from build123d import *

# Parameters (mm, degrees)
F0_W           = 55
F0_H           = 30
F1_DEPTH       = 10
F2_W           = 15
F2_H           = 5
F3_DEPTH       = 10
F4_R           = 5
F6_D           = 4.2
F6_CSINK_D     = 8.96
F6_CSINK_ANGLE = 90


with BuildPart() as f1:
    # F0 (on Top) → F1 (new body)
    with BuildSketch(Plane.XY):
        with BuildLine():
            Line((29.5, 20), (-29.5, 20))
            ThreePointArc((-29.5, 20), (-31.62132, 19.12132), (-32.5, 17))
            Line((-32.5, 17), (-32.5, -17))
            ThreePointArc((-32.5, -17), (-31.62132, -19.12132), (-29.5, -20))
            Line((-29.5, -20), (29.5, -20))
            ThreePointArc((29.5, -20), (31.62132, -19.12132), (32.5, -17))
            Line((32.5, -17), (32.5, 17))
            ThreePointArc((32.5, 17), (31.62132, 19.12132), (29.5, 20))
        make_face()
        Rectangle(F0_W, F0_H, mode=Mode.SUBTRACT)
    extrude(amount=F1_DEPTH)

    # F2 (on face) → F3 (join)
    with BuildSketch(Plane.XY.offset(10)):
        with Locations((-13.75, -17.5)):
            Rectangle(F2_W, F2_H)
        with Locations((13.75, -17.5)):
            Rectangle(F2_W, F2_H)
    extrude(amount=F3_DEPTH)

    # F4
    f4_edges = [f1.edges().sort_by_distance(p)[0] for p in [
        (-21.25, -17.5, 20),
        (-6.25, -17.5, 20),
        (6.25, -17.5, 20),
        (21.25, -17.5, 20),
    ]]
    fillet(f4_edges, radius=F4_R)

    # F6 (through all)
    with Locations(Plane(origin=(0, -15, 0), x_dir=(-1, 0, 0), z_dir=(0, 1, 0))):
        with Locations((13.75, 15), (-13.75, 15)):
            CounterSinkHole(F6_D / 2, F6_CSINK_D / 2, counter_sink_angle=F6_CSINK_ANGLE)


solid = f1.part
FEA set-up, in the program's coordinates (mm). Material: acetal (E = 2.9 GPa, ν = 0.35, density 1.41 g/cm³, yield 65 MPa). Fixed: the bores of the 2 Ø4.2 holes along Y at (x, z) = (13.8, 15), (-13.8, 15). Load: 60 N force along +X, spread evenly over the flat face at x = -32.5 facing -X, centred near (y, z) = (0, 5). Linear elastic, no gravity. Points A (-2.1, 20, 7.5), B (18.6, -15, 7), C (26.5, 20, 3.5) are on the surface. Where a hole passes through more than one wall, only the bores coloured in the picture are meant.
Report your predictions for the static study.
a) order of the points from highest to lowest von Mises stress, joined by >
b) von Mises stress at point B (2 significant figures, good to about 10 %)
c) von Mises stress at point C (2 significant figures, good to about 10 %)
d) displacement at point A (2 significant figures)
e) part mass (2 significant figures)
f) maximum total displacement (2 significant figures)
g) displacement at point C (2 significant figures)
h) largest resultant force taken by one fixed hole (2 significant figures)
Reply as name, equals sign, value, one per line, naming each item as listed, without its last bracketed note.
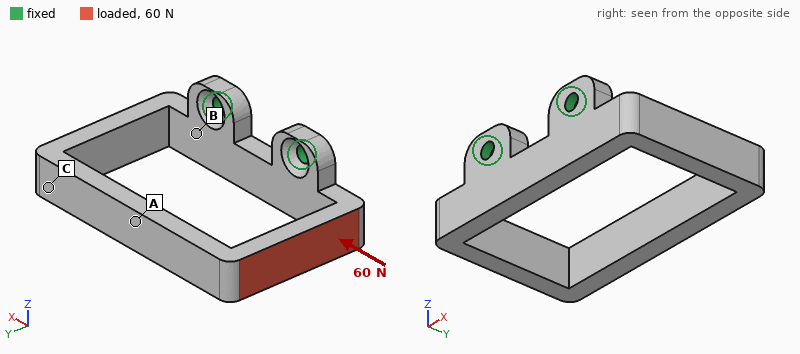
order of the points from highest to lowest von Mises stress, joined by > = B > C > A
von Mises stress at point B = 7.2 MPa
von Mises stress at point C = 4.8 MPa
displacement at point A = 0.79 mm
part mass = 15 g
maximum total displacement = 0.85 mm
displacement at point C = 0.82 mm
largest resultant force taken by one fixed hole = 42 N
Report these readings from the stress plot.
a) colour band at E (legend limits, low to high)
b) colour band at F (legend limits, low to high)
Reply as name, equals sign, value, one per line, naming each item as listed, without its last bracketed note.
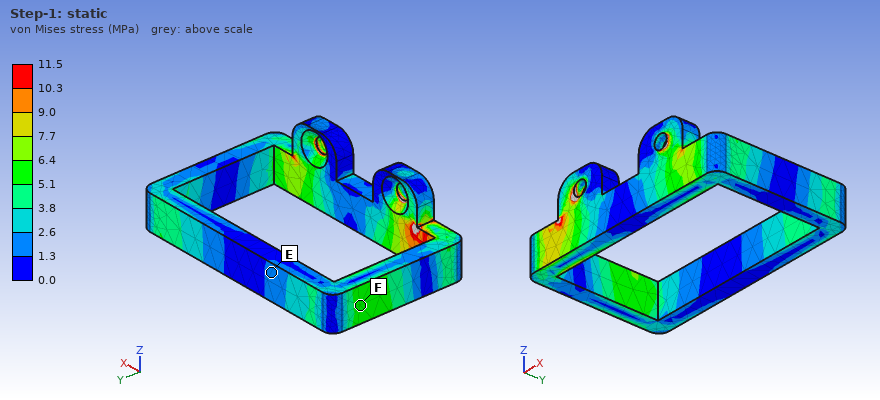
colour band at E = 1.3 to 2.6 MPa
colour band at F = 5.1 to 6.4 MPa
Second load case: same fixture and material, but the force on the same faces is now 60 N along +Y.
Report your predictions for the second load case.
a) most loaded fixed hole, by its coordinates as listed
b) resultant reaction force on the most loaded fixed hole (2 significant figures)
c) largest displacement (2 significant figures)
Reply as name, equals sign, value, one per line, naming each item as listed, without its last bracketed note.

most loaded fixed hole, by its coordinates as listed = (-13.8, 15)
resultant reaction force on the most loaded fixed hole = 80 N
largest displacement = 0.81 mm
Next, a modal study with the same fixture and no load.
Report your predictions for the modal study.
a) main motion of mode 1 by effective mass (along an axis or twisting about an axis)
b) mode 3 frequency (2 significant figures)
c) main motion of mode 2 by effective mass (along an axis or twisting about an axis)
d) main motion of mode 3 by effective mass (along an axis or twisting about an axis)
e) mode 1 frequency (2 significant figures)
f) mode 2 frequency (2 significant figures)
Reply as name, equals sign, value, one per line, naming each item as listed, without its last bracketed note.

main motion of mode 1 by effective mass = along Z
mode 3 frequency = 680 Hz
main motion of mode 2 by effective mass = along X
main motion of mode 3 by effective mass = twisting about Y
mode 1 frequency = 310 Hz
mode 2 frequency = 390 Hz
